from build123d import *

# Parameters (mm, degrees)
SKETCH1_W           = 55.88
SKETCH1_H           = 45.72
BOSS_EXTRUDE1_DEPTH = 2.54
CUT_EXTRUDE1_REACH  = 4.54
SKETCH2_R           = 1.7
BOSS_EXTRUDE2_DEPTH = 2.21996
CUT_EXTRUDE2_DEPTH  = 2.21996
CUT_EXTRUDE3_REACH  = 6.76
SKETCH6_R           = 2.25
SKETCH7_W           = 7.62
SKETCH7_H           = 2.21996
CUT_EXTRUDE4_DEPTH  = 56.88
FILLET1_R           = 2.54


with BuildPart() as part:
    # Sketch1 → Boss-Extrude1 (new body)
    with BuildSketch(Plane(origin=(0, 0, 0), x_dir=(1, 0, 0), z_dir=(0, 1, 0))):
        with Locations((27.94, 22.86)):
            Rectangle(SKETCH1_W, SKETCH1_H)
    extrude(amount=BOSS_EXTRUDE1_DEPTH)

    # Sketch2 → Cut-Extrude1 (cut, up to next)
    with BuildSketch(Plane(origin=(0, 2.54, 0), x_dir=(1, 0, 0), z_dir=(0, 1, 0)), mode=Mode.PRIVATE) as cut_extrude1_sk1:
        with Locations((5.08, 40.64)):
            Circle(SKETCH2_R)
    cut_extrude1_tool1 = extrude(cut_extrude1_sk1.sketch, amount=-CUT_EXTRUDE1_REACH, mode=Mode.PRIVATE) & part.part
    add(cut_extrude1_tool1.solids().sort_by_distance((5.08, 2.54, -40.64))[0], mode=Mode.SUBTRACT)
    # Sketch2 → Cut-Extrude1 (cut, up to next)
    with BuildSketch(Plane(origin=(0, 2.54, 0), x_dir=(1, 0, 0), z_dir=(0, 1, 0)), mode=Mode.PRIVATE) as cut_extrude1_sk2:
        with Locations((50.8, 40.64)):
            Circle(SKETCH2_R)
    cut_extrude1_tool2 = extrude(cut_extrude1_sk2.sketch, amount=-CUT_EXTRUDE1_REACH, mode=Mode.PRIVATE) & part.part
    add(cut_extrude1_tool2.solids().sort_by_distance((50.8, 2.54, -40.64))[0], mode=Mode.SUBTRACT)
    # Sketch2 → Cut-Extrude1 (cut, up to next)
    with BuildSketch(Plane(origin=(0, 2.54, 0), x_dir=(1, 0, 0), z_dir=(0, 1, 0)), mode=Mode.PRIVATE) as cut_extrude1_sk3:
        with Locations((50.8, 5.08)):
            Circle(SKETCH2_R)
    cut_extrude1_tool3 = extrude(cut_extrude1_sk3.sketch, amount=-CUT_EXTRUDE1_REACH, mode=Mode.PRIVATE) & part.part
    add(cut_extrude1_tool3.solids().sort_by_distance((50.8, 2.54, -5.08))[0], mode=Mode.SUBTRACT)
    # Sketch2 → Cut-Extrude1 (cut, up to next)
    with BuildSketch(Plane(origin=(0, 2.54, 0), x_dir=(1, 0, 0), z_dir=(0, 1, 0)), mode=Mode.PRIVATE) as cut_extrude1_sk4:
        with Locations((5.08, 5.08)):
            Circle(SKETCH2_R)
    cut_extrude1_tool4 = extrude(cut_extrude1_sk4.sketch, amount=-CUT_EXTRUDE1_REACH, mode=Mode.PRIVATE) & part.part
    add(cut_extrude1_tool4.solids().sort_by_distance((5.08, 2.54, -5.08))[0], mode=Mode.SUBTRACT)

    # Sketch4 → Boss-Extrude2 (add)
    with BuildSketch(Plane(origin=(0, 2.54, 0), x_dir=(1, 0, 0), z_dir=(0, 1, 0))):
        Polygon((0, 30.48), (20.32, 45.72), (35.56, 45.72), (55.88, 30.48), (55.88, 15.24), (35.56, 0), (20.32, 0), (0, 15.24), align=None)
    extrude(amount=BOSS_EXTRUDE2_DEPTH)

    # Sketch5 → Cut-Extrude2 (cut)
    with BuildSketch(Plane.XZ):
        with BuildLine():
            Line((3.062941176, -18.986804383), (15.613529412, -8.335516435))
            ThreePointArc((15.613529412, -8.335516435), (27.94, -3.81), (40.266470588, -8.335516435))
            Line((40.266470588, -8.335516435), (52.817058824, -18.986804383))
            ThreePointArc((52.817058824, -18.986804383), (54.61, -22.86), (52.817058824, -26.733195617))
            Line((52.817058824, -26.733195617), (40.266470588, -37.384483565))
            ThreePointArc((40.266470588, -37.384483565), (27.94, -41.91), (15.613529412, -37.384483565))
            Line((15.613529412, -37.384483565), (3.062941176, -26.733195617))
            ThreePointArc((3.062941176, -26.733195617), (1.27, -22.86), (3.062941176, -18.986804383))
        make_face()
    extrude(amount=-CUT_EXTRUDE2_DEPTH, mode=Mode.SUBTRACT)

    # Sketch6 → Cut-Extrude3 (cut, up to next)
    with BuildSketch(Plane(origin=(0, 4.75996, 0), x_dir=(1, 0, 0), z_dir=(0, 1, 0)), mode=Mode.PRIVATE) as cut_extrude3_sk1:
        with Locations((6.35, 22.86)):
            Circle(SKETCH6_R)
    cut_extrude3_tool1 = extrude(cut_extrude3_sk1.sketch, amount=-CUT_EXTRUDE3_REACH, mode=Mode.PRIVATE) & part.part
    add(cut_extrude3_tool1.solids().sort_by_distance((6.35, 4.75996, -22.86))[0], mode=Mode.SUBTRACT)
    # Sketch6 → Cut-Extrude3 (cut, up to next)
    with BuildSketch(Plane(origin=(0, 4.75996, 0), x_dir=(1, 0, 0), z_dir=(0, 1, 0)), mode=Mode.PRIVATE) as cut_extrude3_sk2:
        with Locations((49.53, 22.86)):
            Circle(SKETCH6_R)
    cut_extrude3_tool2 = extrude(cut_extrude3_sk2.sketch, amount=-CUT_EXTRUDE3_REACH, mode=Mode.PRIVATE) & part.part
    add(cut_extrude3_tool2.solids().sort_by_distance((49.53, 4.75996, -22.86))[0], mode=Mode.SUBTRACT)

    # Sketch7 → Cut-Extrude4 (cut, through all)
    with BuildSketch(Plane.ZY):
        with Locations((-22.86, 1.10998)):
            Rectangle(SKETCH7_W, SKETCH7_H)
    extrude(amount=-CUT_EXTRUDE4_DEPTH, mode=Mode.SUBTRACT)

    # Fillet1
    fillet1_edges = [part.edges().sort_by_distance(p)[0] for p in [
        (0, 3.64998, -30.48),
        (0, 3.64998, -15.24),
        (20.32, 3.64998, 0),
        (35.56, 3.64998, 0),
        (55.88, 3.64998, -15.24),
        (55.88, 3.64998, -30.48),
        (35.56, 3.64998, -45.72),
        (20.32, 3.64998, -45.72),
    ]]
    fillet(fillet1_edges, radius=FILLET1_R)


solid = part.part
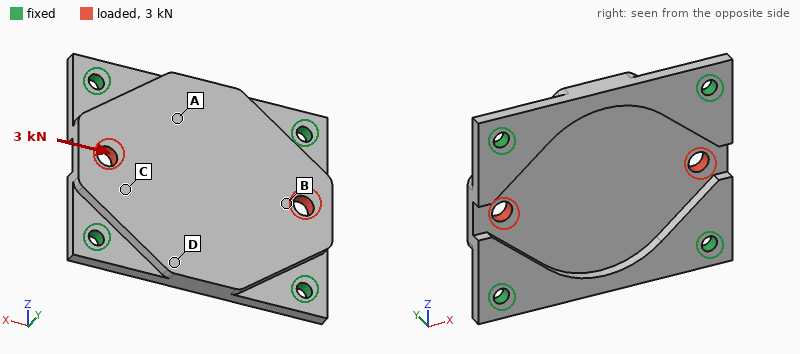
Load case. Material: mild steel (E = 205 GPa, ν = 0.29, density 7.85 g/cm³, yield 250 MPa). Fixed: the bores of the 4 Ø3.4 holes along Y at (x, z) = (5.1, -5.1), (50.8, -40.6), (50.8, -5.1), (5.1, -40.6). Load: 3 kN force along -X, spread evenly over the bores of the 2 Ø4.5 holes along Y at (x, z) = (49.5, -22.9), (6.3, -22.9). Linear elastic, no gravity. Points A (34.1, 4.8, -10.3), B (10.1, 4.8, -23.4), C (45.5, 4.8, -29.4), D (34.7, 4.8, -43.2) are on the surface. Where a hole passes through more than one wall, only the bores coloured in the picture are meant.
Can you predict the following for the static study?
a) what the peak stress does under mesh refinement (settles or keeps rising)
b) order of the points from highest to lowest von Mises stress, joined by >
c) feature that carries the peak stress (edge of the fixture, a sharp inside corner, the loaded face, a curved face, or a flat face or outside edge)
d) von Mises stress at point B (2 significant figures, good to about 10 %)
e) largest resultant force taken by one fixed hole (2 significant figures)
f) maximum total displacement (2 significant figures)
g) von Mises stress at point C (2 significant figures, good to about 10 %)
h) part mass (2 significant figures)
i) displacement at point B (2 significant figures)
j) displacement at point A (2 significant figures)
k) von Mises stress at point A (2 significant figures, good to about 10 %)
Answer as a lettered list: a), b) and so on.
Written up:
a) keeps rising
b) B > C > A > D
c) edge of the fixture
d) 43 MPa
e) 770 N
f) 6.1 µm
g) 30 MPa
h) 59 g
i) 4.7 µm
j) 2.3 µm
k) 15 MPa
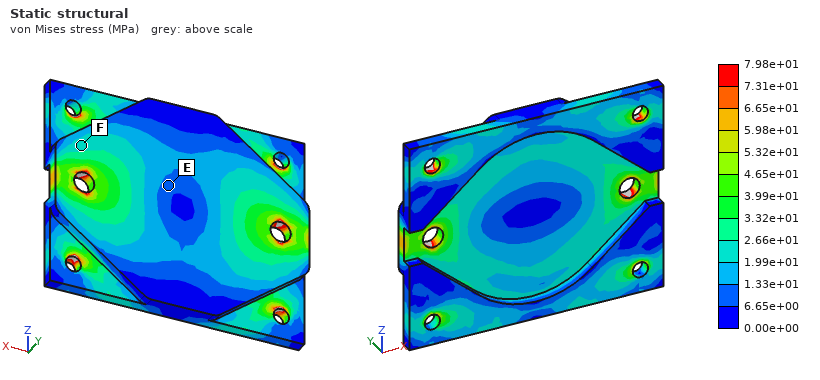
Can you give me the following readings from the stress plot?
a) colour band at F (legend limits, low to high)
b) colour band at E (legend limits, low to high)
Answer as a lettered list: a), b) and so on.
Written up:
a) 1.99e+01 to 2.66e+01 MPa
b) 6.65e+00 to 1.33e+01 MPa
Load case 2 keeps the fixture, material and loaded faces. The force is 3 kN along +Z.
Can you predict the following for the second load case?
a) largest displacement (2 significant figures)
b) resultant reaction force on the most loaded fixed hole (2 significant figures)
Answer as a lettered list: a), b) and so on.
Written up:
a) 3.1 µm
b) 760 N
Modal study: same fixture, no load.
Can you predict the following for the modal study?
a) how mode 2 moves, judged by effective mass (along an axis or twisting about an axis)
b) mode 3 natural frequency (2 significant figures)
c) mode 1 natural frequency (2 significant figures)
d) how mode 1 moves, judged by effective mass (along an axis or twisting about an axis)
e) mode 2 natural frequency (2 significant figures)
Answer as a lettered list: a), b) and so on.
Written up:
a) twisting about X
b) 12 kHz
c) 7400 Hz
d) along Y
e) 9500 Hz
